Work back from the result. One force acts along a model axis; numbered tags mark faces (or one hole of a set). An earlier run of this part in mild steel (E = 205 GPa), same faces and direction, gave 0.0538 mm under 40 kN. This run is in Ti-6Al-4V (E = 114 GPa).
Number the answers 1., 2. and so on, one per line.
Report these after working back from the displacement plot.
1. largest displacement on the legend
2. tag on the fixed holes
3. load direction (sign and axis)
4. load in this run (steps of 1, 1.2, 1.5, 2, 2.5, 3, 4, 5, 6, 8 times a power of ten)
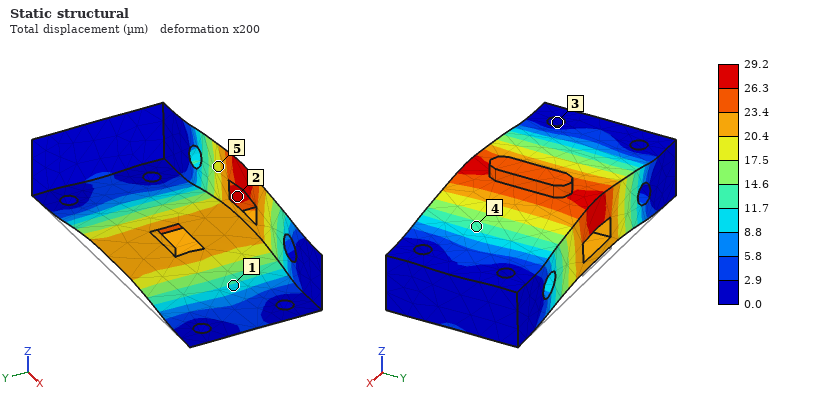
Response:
1. 29.2 µm
2. 3
3. +Z
4. 12 kN
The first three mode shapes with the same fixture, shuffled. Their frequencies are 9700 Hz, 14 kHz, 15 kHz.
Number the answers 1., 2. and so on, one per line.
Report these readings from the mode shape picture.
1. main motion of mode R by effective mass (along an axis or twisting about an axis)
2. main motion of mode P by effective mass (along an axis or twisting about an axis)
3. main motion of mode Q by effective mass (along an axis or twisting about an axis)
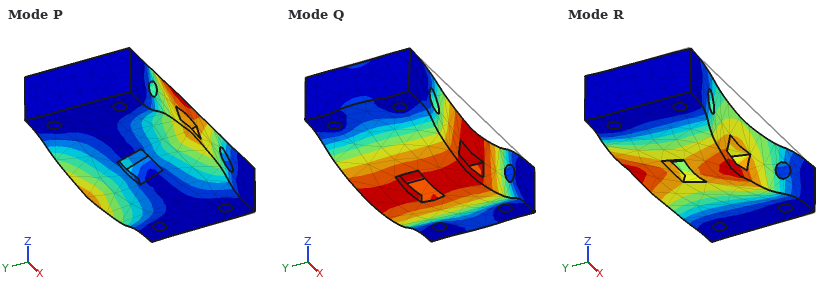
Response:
1. along Y
2. along Y
3. along Z
